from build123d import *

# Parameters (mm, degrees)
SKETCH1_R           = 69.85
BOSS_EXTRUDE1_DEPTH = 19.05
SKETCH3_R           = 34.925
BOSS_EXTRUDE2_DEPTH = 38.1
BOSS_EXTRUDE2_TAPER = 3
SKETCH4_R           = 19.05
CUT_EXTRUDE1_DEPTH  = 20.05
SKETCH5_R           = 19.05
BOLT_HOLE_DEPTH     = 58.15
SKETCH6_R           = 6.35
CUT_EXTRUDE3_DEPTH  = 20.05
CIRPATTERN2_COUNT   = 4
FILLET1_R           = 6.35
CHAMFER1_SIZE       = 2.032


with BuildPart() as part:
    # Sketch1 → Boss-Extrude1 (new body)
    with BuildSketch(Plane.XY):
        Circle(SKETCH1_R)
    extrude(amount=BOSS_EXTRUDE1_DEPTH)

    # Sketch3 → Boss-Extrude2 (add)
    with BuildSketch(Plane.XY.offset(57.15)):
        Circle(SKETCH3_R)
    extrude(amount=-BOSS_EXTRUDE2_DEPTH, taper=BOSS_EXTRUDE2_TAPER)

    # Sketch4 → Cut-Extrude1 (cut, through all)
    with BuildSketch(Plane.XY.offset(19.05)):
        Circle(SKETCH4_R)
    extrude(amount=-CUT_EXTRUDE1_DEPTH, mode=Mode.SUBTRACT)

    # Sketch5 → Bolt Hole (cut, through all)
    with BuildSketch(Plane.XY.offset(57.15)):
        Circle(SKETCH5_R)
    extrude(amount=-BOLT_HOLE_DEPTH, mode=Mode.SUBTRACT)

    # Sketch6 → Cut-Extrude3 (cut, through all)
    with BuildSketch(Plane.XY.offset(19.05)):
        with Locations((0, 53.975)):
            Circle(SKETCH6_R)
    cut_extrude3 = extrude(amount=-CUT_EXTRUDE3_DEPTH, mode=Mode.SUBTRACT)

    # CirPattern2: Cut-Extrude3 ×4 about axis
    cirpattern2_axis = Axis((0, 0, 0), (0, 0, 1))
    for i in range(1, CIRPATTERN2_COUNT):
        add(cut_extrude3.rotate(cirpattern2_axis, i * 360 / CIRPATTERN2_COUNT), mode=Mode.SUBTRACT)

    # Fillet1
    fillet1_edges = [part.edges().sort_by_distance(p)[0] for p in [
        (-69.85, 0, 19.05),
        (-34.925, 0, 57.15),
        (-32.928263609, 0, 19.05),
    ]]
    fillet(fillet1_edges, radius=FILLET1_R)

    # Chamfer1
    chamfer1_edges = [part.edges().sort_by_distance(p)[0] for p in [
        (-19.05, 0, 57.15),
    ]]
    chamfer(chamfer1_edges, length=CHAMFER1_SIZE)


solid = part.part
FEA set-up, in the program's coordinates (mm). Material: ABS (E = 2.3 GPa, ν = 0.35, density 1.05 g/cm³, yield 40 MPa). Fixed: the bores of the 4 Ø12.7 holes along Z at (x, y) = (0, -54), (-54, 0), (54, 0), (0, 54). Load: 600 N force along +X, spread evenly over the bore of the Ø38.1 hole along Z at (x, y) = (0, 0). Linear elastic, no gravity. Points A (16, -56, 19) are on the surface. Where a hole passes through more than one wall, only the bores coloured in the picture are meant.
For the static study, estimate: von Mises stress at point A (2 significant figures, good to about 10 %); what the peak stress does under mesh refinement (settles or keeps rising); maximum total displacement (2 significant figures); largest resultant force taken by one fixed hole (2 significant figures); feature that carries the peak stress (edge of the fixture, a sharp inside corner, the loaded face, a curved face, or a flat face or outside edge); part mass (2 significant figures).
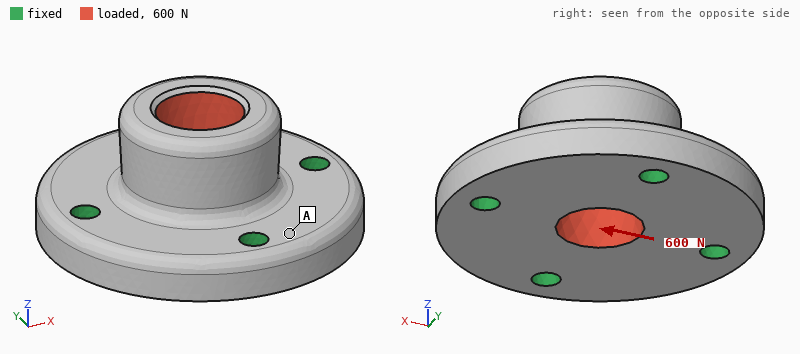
0.14 MPa
keeps rising
17 µm
220 N
edge of the fixture
370 g
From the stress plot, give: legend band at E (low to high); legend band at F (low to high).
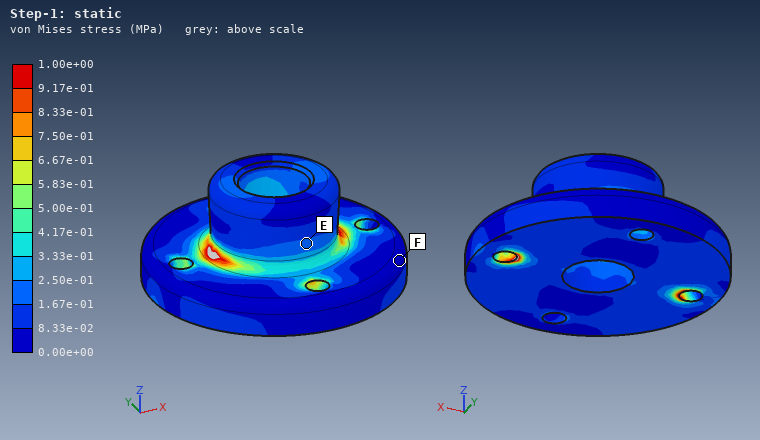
1.67e-01 to 2.50e-01 MPa
0.00e+00 to 8.33e-02 MPa
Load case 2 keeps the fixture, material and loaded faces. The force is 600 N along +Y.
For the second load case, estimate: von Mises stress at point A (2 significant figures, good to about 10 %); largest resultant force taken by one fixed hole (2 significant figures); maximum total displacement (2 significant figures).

0.13 MPa
220 N
17 µm
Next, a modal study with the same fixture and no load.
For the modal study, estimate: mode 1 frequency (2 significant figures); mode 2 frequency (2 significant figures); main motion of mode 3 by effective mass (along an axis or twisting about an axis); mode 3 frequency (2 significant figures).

2600 Hz
2600 Hz
along Z
2800 Hz
